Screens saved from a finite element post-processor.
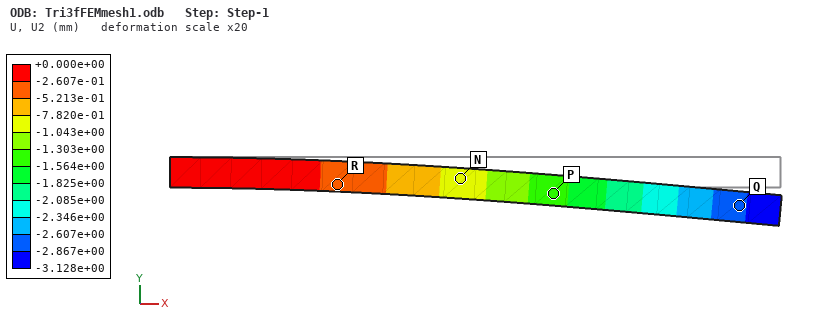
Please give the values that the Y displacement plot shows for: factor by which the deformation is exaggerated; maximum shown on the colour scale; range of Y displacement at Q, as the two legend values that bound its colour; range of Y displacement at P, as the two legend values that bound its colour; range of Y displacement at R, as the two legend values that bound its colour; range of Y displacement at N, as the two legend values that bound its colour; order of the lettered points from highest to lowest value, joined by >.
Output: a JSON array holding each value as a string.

["20", "+0.000e+00 mm", "-2.867e+00 to -2.607e+00 mm", "-1.564e+00 to -1.303e+00 mm", "-5.213e-01 to -2.607e-01 mm", "-1.043e+00 to -7.820e-01 mm", "R > N > P > Q"]
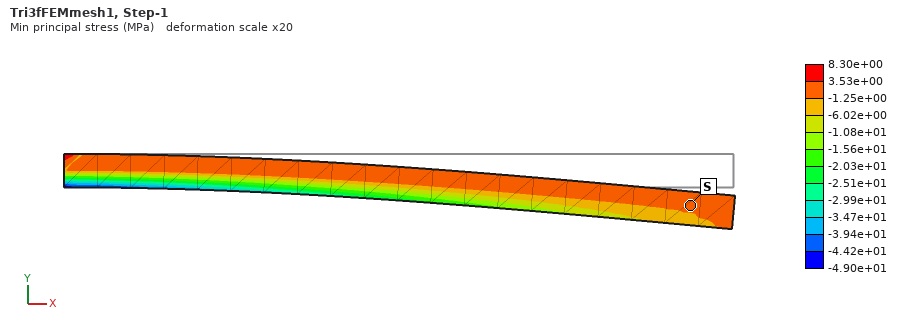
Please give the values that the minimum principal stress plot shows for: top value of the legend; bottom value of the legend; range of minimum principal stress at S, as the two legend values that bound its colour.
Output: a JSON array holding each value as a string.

["8.30e+00 MPa", "-4.90e+01 MPa", "-1.25e+00 to 3.53e+00 MPa"]
